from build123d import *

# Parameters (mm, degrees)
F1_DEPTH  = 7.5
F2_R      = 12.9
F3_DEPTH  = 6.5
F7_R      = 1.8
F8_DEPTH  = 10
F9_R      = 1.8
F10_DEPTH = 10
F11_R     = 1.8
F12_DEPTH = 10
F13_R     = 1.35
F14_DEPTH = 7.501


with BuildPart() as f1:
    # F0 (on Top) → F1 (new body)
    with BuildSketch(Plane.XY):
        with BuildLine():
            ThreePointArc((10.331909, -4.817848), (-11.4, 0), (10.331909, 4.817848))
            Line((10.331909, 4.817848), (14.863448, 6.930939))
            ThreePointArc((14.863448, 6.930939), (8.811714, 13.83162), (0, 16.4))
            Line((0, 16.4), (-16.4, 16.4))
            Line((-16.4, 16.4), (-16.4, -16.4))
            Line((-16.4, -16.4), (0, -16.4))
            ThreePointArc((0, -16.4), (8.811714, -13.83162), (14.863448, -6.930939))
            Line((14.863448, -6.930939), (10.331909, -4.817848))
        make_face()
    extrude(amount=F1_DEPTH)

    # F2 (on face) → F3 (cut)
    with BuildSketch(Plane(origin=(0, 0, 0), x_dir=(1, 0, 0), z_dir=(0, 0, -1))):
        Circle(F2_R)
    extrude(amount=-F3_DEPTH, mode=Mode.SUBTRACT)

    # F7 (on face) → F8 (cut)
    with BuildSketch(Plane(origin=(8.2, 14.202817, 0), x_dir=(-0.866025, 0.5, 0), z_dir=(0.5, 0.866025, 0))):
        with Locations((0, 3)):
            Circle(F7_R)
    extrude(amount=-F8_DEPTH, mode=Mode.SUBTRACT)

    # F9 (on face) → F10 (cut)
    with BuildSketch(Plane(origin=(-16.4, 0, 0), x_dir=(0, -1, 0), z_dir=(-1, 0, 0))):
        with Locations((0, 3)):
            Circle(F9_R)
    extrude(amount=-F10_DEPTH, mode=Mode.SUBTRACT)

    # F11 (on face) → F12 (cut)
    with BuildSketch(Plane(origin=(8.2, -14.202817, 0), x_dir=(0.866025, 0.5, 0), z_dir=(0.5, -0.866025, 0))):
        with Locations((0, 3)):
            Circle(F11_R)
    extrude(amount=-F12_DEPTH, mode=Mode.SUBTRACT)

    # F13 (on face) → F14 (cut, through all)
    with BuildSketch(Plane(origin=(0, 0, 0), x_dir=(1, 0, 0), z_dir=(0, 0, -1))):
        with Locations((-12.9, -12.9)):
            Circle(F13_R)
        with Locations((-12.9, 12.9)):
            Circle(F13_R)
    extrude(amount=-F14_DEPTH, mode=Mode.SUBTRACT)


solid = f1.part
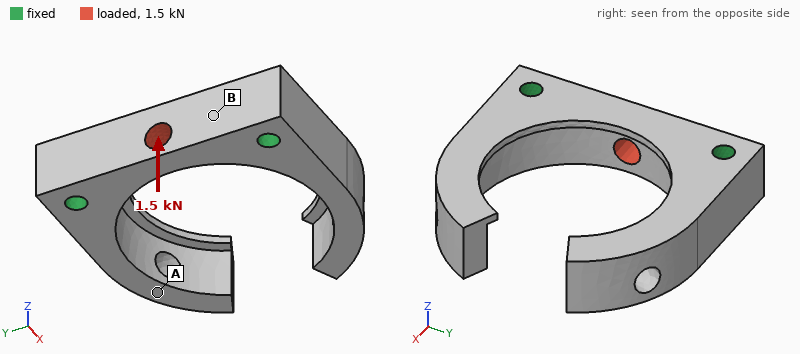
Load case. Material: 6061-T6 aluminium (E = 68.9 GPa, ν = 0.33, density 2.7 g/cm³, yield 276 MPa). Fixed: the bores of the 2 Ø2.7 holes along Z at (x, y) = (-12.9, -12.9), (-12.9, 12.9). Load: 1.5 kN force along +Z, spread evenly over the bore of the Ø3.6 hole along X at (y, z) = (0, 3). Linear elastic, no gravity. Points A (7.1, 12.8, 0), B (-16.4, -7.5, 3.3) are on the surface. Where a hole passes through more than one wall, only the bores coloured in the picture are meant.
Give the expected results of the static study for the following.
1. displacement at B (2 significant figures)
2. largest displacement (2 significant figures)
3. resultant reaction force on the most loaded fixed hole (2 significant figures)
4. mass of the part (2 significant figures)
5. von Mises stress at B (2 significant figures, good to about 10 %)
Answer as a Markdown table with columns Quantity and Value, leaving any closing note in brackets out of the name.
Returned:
| Quantity | Value |
|---|---|
| displacement at B | 7.7 µm |
| largest displacement | 24 µm |
| resultant reaction force on the most loaded fixed hole | 760 N |
| mass of the part | 7.7 g |
| von Mises stress at B | 59 MPa |
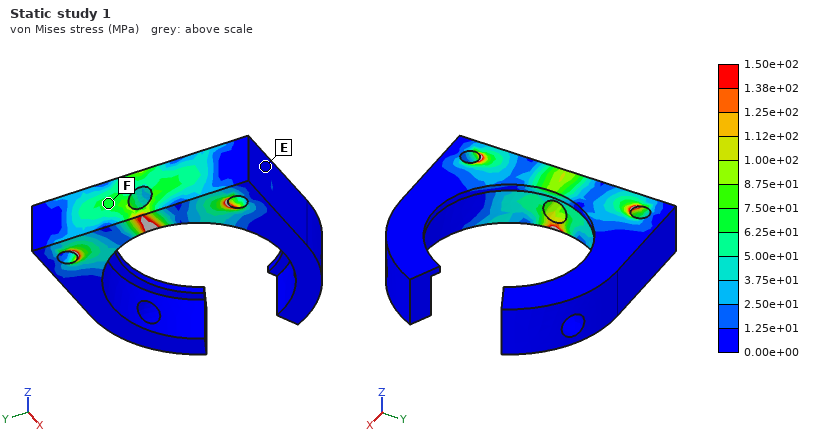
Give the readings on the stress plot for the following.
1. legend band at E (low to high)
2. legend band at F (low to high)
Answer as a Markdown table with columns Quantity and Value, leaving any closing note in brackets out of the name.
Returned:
| Quantity | Value |
|---|---|
| legend band at E | 0.00e+00 to 1.25e+01 MPa |
| legend band at F | 6.25e+01 to 7.50e+01 MPa |
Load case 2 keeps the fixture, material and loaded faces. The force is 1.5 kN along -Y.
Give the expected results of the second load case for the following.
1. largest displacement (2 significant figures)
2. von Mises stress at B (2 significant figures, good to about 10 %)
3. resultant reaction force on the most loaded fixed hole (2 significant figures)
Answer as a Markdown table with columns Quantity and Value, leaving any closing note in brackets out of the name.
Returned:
| Quantity | Value |
|---|---|
| largest displacement | 5.0 µm |
| von Mises stress at B | 22 MPa |
| resultant reaction force on the most loaded fixed hole | 760 N |
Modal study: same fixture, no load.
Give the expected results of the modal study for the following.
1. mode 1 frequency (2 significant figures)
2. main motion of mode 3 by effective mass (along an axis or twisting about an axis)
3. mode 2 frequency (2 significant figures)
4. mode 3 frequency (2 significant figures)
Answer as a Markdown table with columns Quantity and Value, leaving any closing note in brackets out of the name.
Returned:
| Quantity | Value |
|---|---|
| mode 1 frequency | 5800 Hz |
| main motion of mode 3 by effective mass | along Z |
| mode 2 frequency | 6000 Hz |
| mode 3 frequency | 7900 Hz |
